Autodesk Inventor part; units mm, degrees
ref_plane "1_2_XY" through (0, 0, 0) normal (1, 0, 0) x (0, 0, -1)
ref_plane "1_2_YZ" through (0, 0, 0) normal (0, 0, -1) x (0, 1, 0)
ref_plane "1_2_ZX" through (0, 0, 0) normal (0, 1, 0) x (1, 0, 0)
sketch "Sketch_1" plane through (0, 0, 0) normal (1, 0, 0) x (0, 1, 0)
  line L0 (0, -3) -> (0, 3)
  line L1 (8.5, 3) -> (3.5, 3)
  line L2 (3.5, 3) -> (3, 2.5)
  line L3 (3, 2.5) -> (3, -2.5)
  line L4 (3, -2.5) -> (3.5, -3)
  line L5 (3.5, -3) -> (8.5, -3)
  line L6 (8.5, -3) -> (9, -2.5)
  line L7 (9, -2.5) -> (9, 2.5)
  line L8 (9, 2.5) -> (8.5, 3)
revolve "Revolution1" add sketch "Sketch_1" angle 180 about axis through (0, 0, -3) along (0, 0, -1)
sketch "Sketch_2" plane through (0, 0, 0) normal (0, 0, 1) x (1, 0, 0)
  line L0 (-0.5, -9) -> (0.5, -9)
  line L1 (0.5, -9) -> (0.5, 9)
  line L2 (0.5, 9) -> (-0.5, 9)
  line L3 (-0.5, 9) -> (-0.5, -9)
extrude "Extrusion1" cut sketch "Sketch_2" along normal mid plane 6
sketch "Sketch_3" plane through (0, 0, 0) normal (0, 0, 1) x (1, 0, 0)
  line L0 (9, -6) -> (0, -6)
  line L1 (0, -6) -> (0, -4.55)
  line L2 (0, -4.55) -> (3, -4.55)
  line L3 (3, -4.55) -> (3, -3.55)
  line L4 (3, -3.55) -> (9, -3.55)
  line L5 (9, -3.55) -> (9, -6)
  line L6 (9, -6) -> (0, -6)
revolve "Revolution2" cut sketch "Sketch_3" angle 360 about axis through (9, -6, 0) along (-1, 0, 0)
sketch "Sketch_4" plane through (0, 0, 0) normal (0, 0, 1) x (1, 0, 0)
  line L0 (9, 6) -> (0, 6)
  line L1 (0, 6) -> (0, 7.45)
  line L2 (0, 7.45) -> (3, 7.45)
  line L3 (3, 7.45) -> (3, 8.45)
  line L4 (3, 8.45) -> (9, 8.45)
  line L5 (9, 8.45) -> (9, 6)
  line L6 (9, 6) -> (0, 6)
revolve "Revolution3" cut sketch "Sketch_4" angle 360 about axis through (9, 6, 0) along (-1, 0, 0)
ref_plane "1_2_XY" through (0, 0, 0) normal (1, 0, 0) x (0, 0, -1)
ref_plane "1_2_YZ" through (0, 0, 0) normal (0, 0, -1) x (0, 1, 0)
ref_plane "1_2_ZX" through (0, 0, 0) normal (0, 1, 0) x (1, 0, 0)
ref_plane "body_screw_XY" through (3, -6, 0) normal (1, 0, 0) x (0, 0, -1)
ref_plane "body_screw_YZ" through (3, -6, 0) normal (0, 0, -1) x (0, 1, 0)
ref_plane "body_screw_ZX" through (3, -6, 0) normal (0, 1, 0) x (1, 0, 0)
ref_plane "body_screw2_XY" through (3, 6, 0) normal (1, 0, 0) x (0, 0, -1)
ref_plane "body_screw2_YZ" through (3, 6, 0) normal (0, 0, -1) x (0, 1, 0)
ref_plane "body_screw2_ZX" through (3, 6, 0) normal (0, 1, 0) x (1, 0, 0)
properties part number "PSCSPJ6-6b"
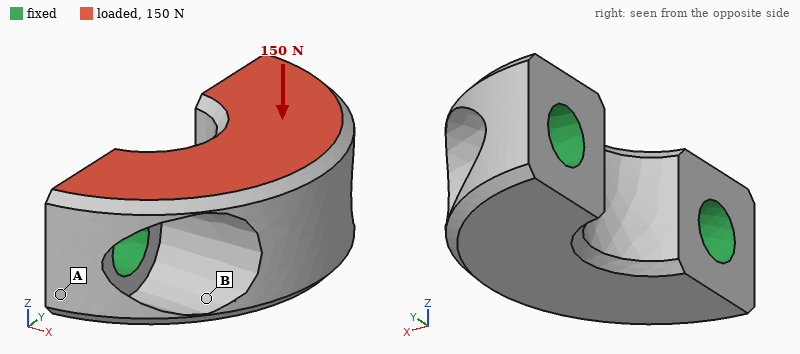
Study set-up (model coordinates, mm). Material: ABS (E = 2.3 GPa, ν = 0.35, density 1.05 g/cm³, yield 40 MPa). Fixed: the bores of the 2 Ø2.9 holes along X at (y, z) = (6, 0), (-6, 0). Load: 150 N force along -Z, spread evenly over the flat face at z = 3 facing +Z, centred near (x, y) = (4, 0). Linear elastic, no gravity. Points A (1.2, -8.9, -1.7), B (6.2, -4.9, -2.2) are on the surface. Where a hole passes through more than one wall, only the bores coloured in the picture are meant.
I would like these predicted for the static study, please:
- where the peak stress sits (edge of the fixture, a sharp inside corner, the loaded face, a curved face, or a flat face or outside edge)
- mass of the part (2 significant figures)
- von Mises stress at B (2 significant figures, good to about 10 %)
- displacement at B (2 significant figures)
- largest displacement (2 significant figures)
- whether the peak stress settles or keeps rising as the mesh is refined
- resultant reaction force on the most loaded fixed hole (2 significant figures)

edge of the fixture
0.49 g
7.0 MPa
58 µm
90 µm
keeps rising
75 N
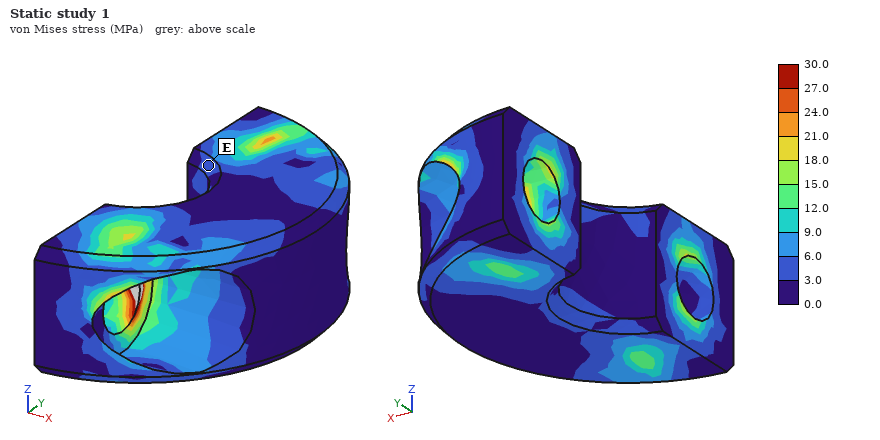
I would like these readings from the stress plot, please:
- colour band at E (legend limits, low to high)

3.0 to 6.0 MPa
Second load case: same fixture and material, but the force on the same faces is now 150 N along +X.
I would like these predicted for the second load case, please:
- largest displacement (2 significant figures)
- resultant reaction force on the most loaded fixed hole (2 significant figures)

76 µm
78 N
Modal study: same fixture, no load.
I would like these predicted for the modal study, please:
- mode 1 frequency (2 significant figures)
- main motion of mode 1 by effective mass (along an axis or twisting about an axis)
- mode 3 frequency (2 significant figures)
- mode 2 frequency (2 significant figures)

11 kHz
along Z
25 kHz
24 kHz
